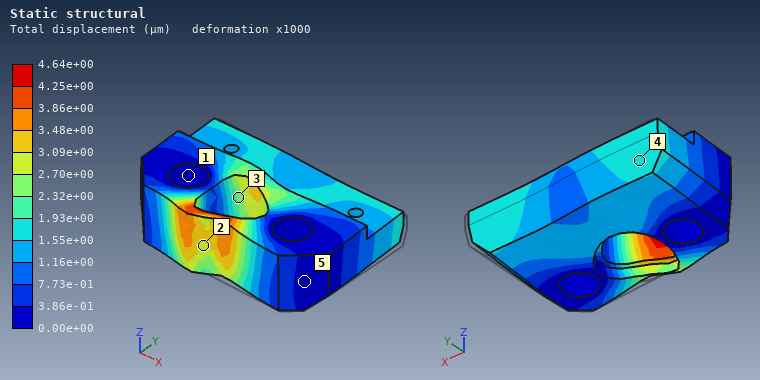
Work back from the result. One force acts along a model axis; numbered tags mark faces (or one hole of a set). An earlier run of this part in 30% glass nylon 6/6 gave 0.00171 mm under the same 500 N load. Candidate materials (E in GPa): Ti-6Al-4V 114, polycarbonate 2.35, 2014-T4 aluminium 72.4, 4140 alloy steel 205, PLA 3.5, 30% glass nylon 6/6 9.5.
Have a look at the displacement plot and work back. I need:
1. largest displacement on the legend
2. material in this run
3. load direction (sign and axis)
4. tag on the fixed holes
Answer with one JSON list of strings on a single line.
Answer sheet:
["4.64e+00 µm", "PLA", "-X", "1"]
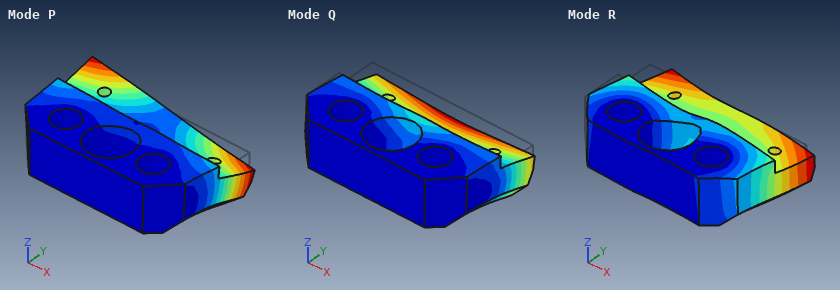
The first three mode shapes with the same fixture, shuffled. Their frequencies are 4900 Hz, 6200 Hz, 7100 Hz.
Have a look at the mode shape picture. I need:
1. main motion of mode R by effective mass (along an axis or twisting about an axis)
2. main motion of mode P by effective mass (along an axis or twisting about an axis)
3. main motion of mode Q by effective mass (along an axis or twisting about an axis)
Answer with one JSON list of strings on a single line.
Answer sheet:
["along X", "twisting about Y", "along Z"]
